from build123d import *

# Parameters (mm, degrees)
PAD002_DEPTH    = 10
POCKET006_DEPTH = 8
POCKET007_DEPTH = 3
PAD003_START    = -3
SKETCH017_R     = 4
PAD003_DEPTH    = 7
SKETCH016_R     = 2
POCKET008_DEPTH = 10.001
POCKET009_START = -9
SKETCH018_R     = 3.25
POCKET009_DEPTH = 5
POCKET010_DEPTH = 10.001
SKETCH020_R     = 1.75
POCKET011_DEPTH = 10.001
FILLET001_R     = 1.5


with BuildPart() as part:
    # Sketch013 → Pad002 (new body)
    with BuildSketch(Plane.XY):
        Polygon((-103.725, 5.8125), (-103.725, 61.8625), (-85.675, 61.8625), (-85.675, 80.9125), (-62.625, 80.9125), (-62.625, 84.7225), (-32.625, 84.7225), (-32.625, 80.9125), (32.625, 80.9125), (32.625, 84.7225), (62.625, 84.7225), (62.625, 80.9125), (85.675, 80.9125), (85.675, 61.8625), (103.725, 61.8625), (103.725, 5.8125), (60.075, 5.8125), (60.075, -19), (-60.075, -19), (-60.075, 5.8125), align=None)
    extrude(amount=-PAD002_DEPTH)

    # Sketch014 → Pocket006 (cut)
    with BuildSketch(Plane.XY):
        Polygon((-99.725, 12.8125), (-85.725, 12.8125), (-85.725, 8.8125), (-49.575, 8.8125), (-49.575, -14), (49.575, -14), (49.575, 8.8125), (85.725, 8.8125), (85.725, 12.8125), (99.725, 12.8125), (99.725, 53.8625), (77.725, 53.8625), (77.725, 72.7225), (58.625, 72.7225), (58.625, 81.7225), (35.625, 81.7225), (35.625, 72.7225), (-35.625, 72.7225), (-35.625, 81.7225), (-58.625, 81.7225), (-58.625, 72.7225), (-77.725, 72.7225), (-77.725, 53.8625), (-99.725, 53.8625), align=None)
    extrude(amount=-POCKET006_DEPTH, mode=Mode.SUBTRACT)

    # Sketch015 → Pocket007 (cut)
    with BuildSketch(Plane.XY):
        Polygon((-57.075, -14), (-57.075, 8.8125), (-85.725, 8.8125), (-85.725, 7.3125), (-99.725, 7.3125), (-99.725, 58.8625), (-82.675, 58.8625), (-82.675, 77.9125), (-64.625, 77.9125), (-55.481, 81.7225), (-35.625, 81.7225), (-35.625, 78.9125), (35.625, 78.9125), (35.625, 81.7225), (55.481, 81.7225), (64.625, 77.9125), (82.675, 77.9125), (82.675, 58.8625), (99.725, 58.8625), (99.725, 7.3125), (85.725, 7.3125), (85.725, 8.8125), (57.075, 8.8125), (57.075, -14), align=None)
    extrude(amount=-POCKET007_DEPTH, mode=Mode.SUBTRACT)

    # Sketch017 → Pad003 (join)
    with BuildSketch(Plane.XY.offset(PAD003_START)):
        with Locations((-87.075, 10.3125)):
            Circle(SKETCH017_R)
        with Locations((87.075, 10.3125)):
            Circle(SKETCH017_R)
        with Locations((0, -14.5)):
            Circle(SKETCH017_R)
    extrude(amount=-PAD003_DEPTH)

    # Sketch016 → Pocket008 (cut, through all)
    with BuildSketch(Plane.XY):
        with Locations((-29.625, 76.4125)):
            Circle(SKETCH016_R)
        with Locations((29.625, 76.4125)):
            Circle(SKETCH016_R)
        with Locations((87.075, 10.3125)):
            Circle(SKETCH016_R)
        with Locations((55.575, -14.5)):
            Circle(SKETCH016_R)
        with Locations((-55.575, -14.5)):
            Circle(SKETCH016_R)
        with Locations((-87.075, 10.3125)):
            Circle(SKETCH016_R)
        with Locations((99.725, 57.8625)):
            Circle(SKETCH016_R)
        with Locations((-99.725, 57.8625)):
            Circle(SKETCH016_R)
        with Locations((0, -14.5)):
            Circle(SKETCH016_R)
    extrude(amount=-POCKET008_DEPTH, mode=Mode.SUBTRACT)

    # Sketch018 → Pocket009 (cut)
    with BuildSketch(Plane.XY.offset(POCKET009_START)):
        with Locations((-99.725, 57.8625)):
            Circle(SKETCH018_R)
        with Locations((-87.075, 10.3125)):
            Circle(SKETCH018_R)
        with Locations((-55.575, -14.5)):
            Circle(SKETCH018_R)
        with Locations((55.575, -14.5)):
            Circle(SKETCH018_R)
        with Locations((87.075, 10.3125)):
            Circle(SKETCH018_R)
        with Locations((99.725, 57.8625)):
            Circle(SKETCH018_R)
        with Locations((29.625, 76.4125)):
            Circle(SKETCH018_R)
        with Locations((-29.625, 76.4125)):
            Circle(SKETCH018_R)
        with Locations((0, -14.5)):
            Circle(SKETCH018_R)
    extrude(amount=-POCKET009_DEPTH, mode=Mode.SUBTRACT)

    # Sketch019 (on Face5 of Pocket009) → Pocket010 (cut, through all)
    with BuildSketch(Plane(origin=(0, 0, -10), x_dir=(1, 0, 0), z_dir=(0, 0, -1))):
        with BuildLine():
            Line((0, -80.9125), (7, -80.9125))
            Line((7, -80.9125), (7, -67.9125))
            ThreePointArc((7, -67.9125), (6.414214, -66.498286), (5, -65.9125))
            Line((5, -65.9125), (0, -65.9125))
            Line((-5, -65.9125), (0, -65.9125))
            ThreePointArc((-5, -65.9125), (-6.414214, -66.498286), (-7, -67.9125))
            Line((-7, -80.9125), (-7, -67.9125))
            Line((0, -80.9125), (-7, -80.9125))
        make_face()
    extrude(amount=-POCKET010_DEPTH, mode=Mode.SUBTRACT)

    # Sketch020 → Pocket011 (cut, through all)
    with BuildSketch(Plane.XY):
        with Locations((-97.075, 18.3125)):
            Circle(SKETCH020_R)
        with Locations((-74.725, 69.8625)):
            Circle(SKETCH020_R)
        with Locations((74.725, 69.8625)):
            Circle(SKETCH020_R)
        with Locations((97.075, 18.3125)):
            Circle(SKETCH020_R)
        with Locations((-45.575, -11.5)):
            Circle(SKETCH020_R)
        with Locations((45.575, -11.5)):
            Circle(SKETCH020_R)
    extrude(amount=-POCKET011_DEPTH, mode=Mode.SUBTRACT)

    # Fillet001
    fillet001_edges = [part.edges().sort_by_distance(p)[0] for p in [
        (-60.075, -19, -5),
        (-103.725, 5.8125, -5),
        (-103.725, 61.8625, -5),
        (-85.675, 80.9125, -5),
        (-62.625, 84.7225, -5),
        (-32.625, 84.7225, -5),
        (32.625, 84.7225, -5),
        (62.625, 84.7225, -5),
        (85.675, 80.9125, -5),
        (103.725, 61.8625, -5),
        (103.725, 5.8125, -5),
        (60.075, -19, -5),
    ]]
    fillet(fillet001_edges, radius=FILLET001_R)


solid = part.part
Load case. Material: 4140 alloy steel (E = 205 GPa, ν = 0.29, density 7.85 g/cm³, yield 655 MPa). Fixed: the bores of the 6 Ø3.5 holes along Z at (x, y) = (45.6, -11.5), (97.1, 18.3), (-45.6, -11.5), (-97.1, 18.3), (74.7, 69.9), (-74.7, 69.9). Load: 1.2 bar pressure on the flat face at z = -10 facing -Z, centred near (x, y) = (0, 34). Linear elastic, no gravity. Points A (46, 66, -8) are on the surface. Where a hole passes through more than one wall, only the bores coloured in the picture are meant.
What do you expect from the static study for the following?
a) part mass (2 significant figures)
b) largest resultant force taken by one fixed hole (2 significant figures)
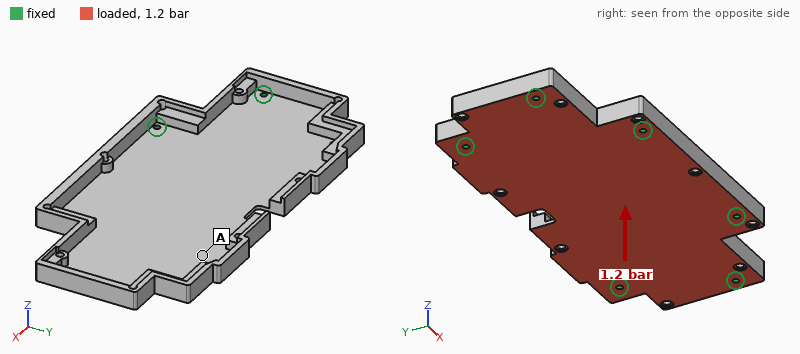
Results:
460 g
690 N
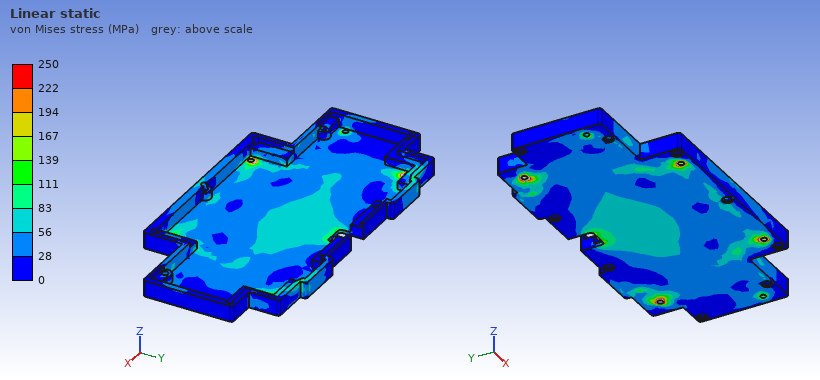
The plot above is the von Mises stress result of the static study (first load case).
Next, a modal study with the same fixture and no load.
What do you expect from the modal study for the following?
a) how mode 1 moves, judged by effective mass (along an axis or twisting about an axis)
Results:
along Z
